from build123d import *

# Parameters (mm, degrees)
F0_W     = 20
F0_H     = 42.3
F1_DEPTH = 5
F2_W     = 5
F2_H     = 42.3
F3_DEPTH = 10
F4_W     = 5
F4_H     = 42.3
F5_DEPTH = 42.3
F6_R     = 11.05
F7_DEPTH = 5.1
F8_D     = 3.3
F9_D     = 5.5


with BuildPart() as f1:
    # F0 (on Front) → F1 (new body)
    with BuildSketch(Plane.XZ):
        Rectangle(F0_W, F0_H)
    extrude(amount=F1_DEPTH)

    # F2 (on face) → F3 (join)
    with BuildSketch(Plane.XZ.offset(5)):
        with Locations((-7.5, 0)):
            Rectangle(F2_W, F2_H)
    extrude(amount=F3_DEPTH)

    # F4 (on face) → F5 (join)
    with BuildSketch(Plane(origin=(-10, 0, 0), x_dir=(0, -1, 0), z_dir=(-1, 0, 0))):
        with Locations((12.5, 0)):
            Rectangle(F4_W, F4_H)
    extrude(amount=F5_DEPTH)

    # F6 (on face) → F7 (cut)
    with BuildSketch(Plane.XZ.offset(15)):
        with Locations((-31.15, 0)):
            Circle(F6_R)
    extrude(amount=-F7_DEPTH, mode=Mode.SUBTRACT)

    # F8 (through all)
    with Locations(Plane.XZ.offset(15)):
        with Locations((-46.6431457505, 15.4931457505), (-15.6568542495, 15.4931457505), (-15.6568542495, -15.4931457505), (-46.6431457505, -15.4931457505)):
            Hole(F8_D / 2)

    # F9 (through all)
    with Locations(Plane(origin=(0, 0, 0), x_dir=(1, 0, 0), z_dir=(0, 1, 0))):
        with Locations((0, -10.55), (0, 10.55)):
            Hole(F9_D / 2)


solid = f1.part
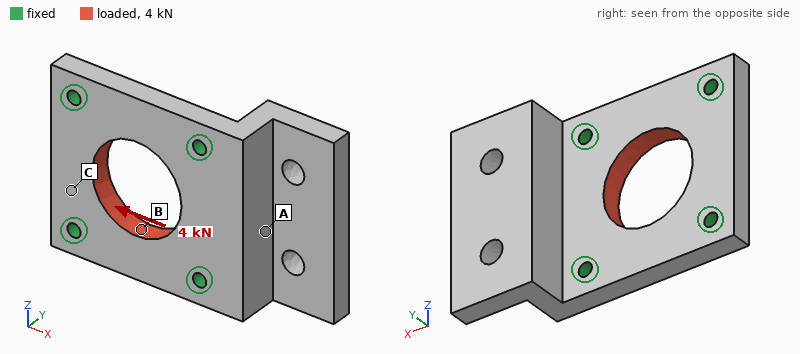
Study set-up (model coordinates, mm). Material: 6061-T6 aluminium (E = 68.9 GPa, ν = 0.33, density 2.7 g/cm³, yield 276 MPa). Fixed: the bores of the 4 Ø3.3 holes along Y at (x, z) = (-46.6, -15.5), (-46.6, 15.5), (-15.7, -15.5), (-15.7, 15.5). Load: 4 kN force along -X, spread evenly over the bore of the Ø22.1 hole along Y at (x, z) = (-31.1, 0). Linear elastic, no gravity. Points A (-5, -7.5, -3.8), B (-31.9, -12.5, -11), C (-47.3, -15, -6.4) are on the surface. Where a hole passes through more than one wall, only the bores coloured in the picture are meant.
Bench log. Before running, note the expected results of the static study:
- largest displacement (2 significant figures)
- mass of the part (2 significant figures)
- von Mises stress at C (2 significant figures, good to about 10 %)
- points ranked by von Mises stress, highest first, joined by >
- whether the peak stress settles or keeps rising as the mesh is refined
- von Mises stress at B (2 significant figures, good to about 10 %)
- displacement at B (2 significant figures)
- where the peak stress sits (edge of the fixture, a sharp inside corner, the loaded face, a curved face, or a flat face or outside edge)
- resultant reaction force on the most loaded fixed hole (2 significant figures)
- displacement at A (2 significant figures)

7.8 µm
35 g
14 MPa
B > C > A
keeps rising
21 MPa
3.3 µm
edge of the fixture
1.0 kN
2.8 µm
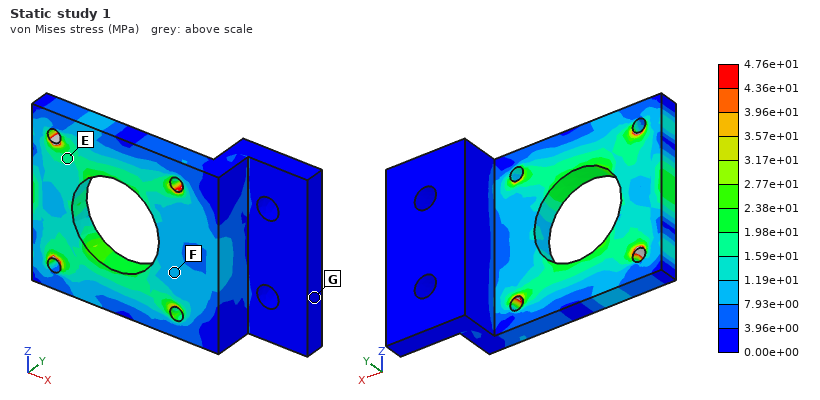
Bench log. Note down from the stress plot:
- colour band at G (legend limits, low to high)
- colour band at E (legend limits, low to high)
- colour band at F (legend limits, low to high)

0.00e+00 to 3.96e+00 MPa
1.59e+01 to 1.98e+01 MPa
7.93e+00 to 1.19e+01 MPa
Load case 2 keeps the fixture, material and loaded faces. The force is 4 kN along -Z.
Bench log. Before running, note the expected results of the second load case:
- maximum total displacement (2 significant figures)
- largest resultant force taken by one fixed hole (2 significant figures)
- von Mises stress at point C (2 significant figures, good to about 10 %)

7.2 µm
1.0 kN
12 MPa
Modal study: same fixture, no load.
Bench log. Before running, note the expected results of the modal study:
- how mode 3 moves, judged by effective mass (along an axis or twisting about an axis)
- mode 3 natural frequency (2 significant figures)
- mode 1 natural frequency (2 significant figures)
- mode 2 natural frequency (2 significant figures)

along Z
15 kHz
4200 Hz
8700 Hz
